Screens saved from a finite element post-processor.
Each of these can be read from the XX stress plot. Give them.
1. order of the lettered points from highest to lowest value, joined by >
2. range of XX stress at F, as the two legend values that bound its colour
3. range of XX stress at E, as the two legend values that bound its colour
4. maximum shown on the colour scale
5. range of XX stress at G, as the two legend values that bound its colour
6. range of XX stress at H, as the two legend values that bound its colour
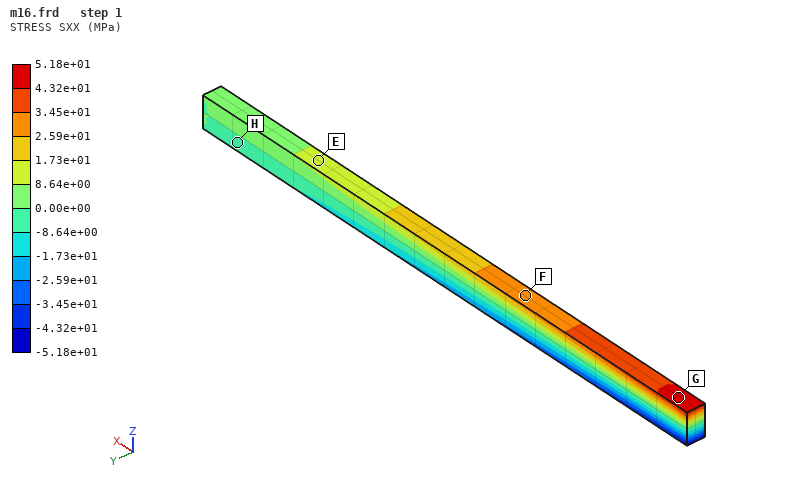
G > F > E > H
2.59e+01 to 3.45e+01 MPa
8.64e+00 to 1.73e+01 MPa
5.18e+01 MPa
4.32e+01 to 5.18e+01 MPa
-8.64e+00 to 0.00e+00 MPa
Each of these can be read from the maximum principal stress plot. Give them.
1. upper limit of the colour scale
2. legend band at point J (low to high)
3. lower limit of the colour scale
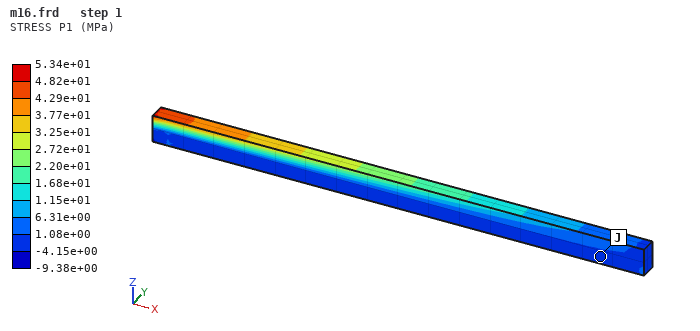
5.34e+01 MPa
-4.15e+00 to 1.08e+00 MPa
-9.38e+00 MPa
